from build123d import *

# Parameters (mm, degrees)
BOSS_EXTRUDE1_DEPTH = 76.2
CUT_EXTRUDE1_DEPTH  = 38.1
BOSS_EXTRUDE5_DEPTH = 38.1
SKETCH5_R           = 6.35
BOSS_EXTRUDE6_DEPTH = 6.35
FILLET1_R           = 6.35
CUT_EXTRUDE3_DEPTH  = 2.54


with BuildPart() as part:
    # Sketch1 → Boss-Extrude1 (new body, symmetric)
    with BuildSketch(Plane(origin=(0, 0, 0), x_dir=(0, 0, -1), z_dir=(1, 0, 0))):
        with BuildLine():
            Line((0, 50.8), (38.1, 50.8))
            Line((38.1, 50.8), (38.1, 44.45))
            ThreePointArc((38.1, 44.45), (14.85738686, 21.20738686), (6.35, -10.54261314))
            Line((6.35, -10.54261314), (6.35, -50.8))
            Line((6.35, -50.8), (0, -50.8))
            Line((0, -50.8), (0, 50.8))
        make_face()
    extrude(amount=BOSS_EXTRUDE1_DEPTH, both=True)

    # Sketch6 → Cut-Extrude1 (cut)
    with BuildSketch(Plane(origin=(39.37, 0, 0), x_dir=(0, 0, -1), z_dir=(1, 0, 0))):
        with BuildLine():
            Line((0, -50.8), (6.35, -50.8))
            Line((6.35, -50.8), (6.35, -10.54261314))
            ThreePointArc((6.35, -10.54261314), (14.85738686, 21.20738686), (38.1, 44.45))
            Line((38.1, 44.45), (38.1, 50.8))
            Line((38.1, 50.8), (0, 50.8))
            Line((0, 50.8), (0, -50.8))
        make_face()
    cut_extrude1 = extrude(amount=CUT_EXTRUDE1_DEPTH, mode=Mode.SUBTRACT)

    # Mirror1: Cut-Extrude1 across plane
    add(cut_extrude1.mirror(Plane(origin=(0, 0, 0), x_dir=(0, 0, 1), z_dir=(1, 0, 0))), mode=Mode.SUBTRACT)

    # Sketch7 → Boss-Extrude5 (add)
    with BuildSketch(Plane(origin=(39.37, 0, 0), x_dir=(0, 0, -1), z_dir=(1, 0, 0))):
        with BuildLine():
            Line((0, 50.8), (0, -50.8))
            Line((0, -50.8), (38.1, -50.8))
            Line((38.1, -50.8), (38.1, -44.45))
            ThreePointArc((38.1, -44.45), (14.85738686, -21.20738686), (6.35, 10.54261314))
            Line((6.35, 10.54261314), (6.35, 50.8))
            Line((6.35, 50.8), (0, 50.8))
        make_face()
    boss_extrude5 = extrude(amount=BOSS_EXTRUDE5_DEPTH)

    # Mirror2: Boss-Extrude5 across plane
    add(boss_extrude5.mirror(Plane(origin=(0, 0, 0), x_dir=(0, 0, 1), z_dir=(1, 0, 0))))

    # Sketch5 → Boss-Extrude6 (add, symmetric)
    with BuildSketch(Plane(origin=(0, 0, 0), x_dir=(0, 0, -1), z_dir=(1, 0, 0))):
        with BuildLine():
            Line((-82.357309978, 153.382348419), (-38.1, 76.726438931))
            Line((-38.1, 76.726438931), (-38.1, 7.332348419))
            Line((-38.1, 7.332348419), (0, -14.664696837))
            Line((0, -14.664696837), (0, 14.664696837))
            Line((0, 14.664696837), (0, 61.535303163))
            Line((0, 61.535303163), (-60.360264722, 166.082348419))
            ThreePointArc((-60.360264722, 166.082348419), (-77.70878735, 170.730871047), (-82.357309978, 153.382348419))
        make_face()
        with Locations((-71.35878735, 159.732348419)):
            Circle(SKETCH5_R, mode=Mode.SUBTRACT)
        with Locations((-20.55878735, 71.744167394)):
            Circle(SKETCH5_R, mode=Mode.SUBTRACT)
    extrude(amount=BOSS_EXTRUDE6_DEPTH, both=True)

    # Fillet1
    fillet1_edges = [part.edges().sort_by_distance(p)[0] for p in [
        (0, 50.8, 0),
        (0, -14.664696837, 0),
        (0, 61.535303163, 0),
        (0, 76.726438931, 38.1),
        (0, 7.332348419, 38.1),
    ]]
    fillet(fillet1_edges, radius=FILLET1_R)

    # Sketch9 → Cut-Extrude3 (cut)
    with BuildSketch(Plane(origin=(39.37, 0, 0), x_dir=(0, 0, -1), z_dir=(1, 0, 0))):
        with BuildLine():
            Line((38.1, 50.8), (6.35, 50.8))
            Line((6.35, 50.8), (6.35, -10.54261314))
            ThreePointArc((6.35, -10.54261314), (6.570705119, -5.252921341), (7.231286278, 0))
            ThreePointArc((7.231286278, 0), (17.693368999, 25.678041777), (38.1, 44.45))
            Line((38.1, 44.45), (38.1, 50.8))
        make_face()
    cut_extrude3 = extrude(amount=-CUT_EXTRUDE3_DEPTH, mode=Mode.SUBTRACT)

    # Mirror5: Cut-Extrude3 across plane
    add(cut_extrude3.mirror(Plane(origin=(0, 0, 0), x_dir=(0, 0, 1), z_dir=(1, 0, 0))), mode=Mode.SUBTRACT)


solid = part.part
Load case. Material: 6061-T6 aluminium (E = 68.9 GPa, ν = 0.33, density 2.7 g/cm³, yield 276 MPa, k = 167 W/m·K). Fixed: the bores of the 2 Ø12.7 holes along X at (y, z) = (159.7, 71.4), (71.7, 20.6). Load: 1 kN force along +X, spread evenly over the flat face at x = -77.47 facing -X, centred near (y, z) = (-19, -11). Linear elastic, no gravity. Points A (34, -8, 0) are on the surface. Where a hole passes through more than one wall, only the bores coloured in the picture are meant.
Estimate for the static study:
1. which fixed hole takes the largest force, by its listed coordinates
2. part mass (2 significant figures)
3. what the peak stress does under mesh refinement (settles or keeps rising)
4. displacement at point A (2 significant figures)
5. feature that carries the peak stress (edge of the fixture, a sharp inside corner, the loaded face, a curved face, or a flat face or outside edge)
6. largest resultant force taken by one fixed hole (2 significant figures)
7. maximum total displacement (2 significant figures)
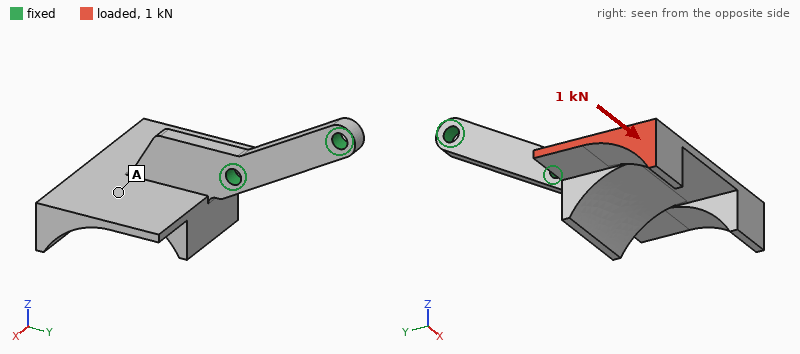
(71.7, 20.6)
740 g
keeps rising
0.44 mm
edge of the fixture
1.0 kN
0.91 mm
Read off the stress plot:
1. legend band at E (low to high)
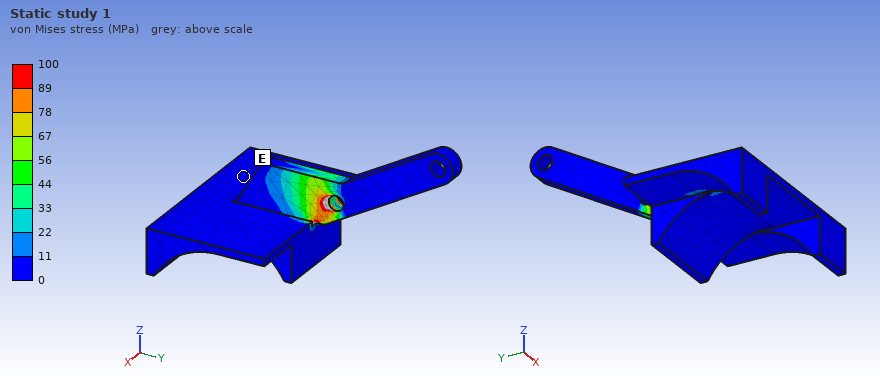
0 to 11 MPa
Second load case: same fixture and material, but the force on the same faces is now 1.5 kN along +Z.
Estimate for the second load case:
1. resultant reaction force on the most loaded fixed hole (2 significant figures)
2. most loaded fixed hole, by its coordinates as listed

1.7 kN
(71.7, 20.6)
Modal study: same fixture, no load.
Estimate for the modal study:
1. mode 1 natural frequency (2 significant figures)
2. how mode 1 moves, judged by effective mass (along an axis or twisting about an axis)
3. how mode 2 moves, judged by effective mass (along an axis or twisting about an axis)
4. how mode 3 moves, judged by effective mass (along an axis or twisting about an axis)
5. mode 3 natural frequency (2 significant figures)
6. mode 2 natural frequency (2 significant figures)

290 Hz
along X
twisting about Y
along Z
550 Hz
460 Hz
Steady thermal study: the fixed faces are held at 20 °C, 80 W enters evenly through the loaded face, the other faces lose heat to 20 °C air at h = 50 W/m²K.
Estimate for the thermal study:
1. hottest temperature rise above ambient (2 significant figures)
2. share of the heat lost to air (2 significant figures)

53 K
65 %
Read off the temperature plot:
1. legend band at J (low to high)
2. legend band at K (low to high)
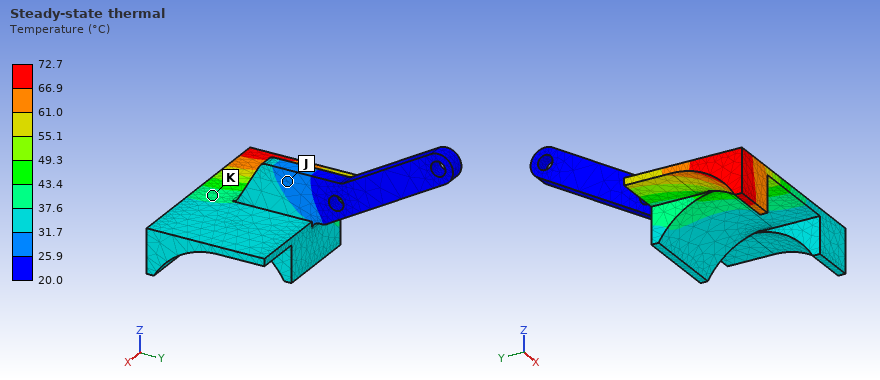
25.9 to 31.7 °C
37.6 to 43.4 °C
